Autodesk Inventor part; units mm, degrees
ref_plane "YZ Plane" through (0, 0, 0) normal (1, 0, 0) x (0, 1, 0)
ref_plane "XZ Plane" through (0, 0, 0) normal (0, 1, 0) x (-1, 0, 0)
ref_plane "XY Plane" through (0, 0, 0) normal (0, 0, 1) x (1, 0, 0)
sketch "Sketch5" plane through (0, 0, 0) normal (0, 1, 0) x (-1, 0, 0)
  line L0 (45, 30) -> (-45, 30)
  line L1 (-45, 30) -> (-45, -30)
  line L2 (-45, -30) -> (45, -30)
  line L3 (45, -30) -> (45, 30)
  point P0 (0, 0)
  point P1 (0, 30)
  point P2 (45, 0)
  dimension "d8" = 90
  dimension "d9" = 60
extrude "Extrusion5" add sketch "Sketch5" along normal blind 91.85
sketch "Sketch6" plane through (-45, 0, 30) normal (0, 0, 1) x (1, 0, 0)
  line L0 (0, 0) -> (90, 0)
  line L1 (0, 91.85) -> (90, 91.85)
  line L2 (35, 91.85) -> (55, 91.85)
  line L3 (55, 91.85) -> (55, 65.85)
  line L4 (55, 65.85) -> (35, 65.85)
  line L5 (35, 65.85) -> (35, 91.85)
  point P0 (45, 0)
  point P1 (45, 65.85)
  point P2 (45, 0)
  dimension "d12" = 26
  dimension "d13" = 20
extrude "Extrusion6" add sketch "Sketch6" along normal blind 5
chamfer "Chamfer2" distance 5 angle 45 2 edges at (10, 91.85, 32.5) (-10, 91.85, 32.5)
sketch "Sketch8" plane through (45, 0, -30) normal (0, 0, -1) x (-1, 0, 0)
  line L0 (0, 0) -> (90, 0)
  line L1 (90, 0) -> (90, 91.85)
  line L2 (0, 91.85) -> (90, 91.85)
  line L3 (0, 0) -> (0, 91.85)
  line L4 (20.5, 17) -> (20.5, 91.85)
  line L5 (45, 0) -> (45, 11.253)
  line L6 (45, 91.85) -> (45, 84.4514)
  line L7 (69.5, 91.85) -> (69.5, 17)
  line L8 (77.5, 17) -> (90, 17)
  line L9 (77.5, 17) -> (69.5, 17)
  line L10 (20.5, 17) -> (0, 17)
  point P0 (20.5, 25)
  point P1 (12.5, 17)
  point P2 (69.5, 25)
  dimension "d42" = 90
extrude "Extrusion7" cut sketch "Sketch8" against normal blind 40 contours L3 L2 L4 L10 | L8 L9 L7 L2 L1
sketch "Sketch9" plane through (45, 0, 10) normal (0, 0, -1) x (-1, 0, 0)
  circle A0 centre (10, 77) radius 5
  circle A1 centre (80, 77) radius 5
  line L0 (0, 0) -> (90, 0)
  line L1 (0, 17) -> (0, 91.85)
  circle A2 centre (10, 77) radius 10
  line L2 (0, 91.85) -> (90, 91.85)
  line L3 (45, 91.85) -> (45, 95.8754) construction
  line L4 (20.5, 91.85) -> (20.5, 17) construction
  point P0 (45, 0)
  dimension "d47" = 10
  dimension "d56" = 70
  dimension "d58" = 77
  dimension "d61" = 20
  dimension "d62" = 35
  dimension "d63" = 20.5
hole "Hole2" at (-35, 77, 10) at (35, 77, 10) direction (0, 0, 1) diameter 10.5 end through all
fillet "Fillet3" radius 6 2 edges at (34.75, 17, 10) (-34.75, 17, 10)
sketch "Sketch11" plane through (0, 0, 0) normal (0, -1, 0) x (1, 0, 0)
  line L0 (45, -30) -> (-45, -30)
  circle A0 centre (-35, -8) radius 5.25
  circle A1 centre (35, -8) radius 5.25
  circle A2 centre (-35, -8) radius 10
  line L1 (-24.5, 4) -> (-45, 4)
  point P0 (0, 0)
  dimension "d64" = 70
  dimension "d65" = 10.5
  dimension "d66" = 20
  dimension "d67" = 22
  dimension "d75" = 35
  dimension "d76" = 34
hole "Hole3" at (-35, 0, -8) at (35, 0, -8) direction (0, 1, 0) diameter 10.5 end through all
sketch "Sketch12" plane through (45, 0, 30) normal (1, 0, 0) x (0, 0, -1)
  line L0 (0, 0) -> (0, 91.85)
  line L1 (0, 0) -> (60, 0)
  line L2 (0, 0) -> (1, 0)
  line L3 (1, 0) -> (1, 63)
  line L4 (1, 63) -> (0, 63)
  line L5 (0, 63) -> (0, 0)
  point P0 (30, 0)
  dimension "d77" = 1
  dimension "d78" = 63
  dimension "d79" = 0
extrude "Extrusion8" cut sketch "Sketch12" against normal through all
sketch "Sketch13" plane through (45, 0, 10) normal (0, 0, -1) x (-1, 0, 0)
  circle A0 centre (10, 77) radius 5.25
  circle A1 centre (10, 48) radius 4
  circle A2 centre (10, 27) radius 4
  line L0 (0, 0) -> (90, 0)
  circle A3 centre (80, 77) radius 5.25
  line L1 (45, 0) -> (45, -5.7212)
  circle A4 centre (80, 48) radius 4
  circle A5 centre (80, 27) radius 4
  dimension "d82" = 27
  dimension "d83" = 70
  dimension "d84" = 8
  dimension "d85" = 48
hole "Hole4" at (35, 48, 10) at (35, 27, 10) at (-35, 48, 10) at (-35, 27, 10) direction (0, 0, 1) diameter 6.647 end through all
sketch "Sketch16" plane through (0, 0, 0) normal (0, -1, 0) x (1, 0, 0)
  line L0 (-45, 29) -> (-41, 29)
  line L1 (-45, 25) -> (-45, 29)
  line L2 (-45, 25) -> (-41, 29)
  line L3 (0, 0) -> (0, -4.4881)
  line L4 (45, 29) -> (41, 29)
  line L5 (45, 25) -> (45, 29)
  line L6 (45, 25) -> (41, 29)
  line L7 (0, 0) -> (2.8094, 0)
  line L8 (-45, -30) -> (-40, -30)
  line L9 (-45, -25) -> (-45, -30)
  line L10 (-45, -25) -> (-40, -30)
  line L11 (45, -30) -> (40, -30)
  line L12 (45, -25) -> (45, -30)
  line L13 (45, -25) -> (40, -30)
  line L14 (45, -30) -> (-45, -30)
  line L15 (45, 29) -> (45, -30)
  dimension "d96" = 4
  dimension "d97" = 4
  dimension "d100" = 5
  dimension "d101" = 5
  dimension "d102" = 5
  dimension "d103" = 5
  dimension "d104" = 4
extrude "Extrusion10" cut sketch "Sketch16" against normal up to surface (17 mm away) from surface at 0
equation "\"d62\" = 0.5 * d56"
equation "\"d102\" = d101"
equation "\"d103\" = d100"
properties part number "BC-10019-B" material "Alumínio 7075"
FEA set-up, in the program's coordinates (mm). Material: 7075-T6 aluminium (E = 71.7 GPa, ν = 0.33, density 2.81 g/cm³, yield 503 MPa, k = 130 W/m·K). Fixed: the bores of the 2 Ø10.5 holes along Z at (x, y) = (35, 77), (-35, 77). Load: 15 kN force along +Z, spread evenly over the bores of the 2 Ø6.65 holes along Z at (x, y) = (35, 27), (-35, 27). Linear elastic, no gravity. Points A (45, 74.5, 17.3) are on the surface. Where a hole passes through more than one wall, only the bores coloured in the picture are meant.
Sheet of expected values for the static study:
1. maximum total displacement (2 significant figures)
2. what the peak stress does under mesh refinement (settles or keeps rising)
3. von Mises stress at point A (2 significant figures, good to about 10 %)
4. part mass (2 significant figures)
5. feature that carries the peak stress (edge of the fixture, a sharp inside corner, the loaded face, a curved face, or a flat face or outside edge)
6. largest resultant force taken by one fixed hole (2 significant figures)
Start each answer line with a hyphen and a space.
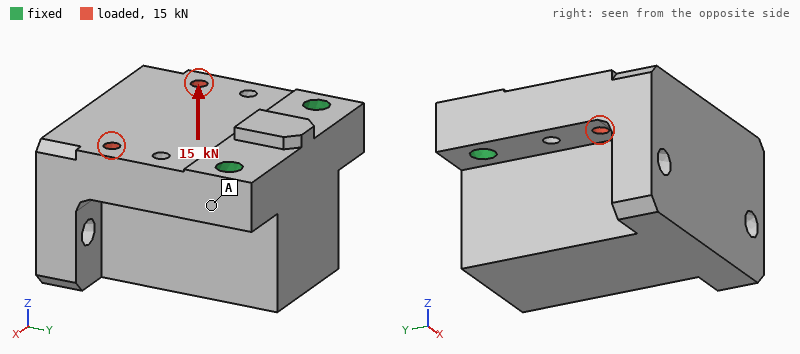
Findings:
- 0.26 mm
- keeps rising
- 33 MPa
- 1.0 kg
- edge of the fixture
- 7.6 kN
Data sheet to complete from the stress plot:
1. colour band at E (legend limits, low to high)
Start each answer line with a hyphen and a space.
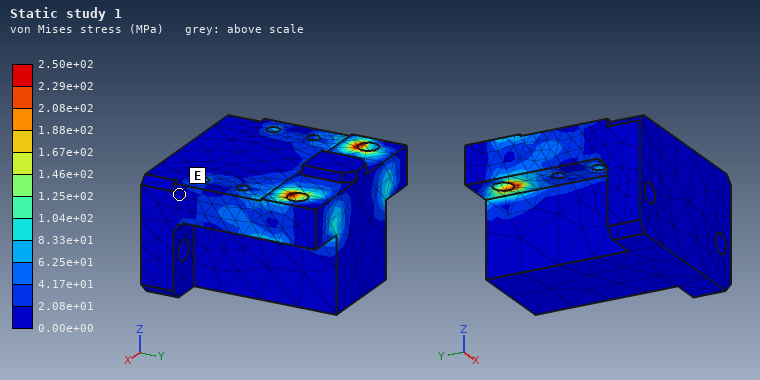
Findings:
- 0.00e+00 to 2.08e+01 MPa
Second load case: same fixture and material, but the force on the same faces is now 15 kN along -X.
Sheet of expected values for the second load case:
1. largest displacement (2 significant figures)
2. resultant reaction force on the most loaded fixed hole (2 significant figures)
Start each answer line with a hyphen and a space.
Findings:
- 34 µm
- 13 kN
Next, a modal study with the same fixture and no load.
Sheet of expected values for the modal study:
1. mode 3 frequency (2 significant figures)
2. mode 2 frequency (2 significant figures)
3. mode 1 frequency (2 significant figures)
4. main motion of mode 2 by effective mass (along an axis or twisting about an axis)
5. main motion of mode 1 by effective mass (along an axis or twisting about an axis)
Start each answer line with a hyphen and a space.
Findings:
- 6000 Hz
- 4300 Hz
- 1600 Hz
- along X
- along Z
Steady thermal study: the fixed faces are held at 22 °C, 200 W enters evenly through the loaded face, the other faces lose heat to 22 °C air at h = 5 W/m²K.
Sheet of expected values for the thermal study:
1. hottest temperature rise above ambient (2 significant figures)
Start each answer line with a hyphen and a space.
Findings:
- 49 K
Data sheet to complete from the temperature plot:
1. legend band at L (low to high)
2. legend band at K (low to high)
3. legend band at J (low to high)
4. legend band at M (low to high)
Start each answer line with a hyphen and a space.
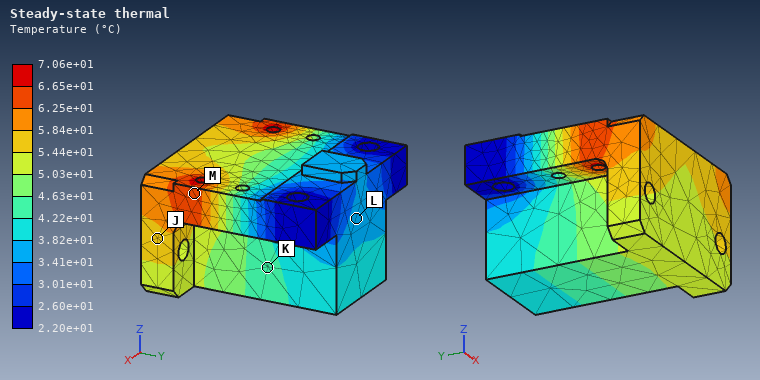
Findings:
- 3.41e+01 to 3.82e+01 °C
- 4.22e+01 to 4.63e+01 °C
- 5.44e+01 to 5.84e+01 °C
- 6.25e+01 to 6.65e+01 °C
